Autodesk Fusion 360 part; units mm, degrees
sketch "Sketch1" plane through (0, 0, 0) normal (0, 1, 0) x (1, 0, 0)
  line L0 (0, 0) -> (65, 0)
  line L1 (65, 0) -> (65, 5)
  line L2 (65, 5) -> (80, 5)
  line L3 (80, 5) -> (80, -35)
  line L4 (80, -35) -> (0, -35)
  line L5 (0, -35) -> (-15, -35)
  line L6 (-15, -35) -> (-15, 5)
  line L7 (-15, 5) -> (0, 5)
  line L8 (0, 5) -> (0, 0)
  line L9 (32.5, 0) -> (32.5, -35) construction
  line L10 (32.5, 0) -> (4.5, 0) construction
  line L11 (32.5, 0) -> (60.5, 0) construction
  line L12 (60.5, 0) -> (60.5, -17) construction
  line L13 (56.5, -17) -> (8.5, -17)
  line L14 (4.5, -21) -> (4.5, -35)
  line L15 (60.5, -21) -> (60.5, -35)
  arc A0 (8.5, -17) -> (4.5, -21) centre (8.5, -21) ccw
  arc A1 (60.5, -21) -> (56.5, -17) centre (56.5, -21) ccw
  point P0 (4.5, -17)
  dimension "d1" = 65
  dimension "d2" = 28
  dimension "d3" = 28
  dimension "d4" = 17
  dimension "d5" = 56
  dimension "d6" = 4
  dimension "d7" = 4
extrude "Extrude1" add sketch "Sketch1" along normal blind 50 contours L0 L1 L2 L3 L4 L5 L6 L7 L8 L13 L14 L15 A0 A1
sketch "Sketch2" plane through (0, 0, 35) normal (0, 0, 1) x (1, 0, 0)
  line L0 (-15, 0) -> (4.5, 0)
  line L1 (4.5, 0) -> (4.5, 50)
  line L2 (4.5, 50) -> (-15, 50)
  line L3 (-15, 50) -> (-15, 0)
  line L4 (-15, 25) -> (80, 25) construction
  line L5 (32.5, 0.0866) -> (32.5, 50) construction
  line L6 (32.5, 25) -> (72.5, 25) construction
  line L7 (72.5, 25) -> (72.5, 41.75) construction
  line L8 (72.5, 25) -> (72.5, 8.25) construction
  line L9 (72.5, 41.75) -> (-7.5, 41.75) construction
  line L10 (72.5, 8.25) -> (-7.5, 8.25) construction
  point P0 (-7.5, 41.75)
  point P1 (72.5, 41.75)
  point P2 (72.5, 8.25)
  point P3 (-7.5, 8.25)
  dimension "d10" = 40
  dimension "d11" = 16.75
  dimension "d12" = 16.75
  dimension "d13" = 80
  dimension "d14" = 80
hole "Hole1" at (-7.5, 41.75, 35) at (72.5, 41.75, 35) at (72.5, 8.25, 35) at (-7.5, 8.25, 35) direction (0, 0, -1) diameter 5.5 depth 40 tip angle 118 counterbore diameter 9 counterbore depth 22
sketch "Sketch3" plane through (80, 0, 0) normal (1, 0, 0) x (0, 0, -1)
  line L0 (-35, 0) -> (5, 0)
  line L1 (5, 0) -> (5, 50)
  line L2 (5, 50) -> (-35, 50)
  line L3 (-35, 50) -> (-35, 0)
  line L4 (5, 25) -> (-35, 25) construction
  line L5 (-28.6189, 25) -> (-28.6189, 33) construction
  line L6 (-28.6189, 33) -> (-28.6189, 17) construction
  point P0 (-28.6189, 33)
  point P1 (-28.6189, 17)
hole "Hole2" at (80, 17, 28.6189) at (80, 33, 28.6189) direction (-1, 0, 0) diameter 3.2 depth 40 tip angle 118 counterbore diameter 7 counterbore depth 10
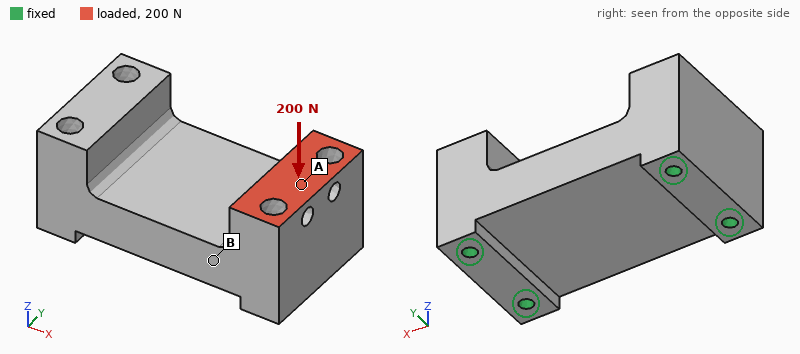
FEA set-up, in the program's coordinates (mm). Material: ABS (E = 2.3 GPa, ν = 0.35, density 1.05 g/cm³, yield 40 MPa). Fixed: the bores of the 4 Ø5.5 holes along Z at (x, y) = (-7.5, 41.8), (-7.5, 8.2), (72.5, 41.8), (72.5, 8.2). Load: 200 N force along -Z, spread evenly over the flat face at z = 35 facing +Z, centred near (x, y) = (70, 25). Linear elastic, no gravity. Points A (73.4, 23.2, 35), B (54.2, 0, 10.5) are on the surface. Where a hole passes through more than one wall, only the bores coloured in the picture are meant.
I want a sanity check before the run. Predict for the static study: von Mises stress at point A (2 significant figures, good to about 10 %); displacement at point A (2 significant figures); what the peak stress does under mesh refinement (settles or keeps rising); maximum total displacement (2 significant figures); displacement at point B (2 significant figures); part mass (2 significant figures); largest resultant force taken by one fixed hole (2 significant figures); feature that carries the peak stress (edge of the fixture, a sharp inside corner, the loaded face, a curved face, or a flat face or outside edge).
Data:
0.35 MPa
4.5 µm
keeps rising
5.7 µm
2.3 µm
120 g
99 N
edge of the fixture
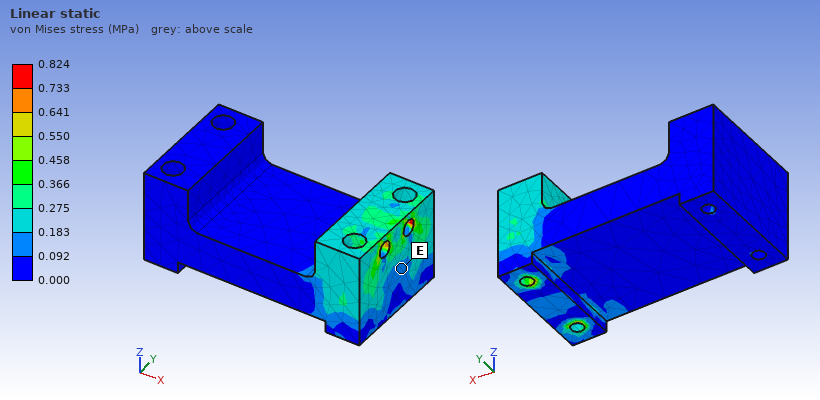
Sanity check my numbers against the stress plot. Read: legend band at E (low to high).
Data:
0.092 to 0.183 MPa
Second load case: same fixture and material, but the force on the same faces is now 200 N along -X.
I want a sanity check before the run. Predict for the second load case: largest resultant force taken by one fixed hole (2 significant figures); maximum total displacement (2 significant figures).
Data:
61 N
44 µm
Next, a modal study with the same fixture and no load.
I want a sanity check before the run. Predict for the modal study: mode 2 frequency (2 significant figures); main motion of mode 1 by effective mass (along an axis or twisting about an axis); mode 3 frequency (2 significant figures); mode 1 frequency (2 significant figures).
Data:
4100 Hz
along Z
4200 Hz
2700 Hz
